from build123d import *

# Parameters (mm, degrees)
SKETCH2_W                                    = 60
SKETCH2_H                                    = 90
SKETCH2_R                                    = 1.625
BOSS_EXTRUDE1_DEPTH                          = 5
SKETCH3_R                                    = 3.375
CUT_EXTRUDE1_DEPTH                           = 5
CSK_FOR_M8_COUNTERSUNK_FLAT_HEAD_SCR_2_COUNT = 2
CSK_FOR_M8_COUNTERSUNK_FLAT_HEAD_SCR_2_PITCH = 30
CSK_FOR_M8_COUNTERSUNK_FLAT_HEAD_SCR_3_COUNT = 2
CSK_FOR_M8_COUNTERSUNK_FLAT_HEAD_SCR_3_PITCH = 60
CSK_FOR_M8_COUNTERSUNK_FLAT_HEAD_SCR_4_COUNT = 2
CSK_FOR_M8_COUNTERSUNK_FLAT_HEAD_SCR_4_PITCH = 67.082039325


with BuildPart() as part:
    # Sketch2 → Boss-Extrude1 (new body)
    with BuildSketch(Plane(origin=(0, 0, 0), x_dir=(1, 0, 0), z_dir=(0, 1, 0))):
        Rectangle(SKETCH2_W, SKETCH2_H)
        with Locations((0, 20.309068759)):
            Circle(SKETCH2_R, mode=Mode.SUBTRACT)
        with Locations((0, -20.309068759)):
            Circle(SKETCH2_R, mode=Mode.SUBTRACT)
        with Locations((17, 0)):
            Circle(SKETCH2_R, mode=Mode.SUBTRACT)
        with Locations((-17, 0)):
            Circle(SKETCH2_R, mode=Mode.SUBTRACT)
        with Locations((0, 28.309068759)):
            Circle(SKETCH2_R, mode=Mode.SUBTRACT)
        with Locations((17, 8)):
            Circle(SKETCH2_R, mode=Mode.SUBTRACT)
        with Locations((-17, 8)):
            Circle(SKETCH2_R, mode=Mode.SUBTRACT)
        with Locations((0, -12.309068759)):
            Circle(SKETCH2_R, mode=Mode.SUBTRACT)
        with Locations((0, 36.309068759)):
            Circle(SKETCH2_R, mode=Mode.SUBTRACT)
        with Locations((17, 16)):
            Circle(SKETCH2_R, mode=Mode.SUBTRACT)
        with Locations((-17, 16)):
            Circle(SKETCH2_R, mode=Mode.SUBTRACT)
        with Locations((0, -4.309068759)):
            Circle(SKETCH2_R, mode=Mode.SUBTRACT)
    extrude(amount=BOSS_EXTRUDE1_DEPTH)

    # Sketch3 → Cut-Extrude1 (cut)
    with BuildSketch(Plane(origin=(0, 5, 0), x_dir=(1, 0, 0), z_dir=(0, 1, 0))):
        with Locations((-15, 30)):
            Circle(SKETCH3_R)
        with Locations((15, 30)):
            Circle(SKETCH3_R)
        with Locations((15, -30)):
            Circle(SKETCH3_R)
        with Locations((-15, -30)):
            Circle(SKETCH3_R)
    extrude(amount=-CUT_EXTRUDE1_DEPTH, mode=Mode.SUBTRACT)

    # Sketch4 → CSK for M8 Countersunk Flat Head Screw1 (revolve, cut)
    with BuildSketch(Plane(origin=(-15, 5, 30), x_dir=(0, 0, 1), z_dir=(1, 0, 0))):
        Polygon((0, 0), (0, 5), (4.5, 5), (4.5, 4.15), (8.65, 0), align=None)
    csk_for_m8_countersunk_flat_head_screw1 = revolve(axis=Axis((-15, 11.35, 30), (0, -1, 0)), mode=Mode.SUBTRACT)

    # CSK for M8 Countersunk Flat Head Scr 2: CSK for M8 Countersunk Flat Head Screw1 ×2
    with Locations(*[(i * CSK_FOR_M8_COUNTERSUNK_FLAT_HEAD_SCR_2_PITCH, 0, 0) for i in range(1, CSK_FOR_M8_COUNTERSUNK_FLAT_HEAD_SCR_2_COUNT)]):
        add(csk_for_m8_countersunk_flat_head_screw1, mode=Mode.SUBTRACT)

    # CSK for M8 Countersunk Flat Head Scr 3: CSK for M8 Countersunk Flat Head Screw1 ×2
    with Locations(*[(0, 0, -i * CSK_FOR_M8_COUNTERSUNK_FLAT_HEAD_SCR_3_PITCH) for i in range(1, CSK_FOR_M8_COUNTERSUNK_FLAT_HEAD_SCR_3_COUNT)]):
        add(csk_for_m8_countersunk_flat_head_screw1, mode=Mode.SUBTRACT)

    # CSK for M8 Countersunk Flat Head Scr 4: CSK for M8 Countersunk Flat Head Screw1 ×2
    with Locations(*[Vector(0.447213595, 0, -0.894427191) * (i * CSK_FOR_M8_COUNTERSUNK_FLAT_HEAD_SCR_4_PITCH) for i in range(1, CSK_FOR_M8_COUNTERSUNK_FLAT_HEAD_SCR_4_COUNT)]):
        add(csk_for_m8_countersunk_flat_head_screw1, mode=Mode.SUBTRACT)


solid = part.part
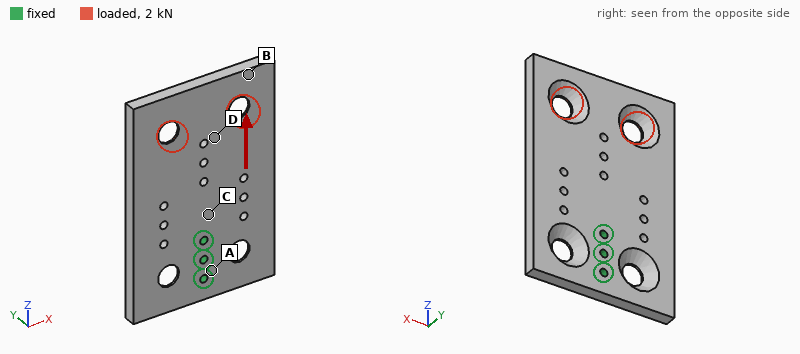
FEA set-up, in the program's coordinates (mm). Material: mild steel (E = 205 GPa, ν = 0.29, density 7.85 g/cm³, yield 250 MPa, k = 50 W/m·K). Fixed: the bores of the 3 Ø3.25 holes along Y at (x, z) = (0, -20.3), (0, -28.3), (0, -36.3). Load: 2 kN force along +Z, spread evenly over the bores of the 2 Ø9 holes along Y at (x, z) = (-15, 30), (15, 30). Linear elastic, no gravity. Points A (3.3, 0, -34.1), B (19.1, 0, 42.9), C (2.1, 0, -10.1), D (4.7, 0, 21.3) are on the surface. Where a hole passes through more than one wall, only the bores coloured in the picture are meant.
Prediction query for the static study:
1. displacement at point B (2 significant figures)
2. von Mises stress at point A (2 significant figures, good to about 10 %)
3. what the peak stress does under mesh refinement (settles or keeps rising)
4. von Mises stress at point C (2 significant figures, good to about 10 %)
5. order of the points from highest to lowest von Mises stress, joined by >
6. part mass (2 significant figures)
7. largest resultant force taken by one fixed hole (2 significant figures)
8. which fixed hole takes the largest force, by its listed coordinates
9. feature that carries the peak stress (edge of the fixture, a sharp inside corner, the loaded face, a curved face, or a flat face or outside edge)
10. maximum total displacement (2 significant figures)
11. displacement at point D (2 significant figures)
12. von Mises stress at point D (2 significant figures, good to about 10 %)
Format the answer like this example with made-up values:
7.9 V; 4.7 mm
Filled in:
76 µm; 9.6 MPa; keeps rising; 33 MPa; C > D > A > B; 190 g; 1.2 kN; (0, -20.3); edge of the fixture; 81 µm; 37 µm; 25 MPa
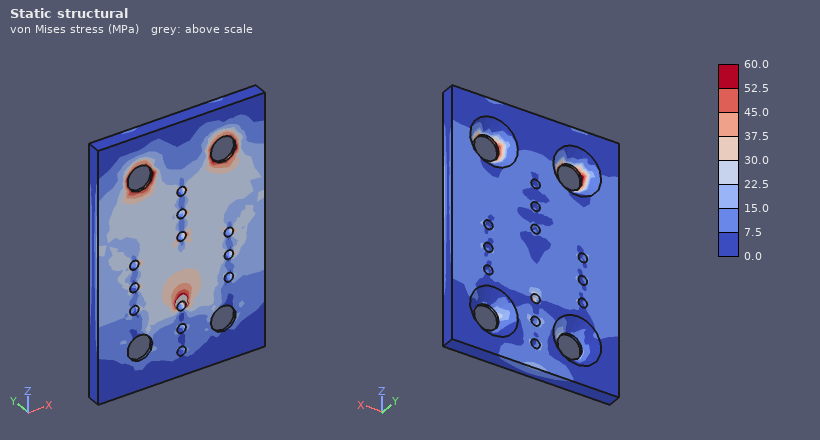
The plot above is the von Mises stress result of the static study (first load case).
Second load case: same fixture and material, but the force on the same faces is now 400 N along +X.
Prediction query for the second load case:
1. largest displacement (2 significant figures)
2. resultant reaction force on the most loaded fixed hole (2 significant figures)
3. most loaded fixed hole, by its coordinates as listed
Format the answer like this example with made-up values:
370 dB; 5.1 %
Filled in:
19 µm; 1.5 kN; (0, -20.3)
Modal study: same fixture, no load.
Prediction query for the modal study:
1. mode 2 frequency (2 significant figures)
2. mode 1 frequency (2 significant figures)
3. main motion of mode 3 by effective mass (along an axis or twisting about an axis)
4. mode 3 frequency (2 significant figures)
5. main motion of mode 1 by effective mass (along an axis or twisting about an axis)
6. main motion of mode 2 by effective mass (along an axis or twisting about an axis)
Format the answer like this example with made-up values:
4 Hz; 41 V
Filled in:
1700 Hz; 870 Hz; along X; 3100 Hz; along Y; twisting about Z
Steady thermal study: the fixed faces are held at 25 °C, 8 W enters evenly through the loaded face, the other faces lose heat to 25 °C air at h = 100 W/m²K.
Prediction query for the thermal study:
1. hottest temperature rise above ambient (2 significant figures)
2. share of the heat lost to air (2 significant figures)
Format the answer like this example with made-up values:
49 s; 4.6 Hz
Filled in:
17 K; 82 %
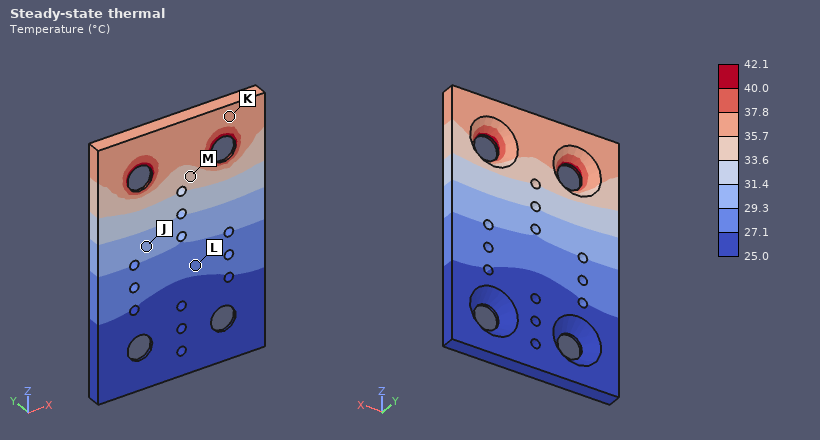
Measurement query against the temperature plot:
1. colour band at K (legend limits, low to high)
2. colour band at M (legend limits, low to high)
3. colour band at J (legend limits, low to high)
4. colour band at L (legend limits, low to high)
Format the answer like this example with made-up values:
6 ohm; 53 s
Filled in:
35.7 to 37.8 °C; 33.6 to 35.7 °C; 29.3 to 31.4 °C; 27.1 to 29.3 °C
